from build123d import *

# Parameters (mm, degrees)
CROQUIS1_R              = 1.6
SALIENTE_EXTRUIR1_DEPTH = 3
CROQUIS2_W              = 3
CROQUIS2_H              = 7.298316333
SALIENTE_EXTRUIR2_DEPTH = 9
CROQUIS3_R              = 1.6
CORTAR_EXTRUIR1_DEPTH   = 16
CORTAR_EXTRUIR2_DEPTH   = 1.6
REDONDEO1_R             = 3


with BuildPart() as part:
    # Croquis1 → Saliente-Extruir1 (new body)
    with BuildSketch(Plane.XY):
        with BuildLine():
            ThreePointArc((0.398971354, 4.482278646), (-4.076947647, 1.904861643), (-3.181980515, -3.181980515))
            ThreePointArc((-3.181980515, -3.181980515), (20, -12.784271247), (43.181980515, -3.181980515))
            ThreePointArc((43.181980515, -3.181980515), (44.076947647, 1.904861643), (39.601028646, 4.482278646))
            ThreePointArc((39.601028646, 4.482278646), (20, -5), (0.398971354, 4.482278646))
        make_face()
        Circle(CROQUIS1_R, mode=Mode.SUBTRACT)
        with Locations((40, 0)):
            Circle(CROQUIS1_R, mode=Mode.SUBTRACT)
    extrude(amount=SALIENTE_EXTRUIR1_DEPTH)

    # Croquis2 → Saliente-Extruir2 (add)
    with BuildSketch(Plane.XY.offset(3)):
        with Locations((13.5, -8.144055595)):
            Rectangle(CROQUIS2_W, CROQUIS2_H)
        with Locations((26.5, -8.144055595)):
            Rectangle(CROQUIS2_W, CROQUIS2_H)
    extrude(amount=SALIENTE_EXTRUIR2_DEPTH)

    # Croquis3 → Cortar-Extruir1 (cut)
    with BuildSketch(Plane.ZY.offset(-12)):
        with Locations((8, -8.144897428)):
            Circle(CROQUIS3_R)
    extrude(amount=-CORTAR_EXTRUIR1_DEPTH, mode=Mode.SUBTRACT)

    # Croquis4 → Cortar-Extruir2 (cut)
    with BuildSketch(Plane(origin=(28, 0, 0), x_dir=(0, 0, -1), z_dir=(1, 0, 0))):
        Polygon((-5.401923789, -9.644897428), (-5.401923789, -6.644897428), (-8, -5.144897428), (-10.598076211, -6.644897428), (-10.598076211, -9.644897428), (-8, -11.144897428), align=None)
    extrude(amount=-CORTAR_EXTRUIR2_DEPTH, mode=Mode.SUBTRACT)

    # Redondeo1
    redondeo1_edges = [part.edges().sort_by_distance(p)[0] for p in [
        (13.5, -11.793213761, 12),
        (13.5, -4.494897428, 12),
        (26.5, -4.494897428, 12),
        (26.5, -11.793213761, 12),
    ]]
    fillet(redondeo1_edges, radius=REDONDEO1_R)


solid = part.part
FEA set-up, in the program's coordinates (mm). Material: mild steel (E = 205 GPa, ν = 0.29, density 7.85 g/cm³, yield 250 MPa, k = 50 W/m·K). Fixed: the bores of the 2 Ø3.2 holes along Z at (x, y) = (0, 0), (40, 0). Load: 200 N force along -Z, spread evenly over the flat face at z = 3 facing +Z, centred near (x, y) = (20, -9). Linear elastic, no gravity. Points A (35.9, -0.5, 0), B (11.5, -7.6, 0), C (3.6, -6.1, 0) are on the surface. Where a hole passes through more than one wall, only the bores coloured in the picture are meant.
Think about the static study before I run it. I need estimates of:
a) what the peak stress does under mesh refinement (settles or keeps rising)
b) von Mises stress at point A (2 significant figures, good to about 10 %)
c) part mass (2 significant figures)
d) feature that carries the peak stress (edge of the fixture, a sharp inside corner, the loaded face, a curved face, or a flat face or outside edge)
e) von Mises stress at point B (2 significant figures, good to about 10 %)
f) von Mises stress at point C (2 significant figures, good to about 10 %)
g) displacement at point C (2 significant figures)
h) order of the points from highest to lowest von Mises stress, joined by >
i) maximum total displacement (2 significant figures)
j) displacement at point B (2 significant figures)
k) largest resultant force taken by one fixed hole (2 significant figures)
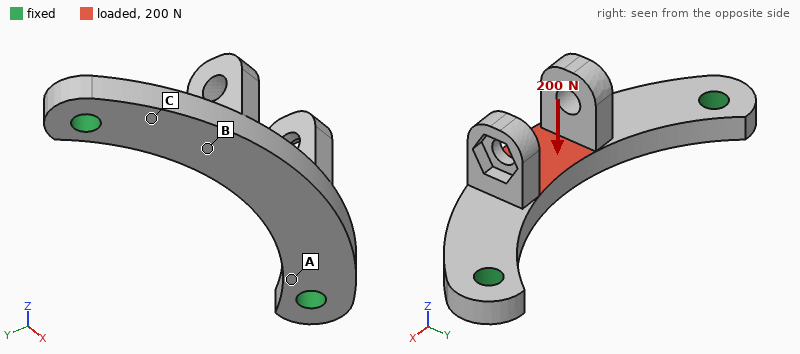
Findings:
keeps rising
78 MPa
12 g
edge of the fixture
22 MPa
53 MPa
5.7 µm
A > C > B
34 µm
18 µm
100 N
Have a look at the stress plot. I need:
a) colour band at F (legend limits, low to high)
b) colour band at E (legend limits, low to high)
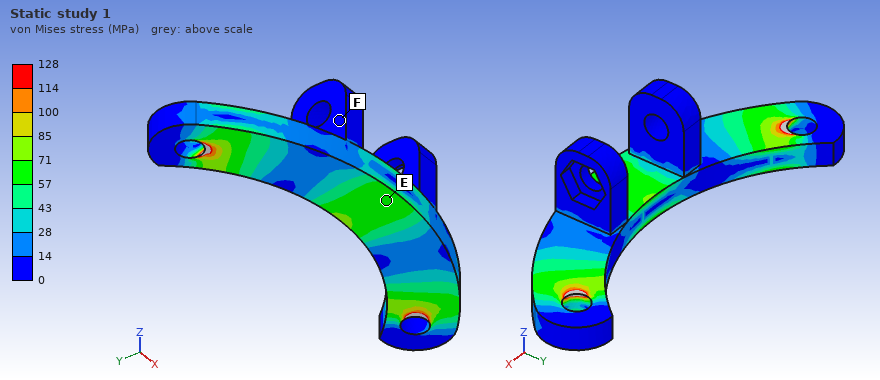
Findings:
0 to 14 MPa
57 to 71 MPa
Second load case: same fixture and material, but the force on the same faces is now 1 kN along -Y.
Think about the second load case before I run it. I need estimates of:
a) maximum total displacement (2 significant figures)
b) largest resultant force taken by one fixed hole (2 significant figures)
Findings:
37 µm
830 N
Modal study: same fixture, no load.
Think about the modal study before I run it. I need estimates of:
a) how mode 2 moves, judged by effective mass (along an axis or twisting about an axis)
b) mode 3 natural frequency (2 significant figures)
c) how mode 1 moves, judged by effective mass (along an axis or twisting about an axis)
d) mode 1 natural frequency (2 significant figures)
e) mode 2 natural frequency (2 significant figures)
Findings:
along Y
15 kHz
along Z
5800 Hz
12 kHz
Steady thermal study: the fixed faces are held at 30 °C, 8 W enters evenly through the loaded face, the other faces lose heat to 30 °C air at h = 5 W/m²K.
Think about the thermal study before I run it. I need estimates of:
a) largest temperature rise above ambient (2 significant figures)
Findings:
65 K
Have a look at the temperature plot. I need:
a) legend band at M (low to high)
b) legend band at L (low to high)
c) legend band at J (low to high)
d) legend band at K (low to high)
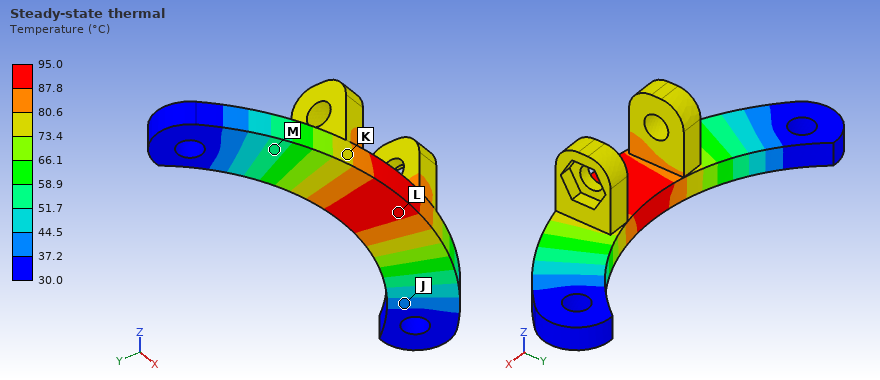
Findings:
51.7 to 58.9 °C
87.8 to 95.0 °C
37.2 to 44.5 °C
73.4 to 80.6 °C
